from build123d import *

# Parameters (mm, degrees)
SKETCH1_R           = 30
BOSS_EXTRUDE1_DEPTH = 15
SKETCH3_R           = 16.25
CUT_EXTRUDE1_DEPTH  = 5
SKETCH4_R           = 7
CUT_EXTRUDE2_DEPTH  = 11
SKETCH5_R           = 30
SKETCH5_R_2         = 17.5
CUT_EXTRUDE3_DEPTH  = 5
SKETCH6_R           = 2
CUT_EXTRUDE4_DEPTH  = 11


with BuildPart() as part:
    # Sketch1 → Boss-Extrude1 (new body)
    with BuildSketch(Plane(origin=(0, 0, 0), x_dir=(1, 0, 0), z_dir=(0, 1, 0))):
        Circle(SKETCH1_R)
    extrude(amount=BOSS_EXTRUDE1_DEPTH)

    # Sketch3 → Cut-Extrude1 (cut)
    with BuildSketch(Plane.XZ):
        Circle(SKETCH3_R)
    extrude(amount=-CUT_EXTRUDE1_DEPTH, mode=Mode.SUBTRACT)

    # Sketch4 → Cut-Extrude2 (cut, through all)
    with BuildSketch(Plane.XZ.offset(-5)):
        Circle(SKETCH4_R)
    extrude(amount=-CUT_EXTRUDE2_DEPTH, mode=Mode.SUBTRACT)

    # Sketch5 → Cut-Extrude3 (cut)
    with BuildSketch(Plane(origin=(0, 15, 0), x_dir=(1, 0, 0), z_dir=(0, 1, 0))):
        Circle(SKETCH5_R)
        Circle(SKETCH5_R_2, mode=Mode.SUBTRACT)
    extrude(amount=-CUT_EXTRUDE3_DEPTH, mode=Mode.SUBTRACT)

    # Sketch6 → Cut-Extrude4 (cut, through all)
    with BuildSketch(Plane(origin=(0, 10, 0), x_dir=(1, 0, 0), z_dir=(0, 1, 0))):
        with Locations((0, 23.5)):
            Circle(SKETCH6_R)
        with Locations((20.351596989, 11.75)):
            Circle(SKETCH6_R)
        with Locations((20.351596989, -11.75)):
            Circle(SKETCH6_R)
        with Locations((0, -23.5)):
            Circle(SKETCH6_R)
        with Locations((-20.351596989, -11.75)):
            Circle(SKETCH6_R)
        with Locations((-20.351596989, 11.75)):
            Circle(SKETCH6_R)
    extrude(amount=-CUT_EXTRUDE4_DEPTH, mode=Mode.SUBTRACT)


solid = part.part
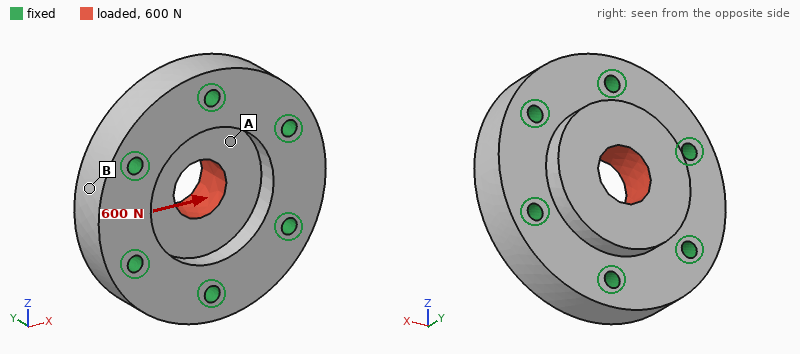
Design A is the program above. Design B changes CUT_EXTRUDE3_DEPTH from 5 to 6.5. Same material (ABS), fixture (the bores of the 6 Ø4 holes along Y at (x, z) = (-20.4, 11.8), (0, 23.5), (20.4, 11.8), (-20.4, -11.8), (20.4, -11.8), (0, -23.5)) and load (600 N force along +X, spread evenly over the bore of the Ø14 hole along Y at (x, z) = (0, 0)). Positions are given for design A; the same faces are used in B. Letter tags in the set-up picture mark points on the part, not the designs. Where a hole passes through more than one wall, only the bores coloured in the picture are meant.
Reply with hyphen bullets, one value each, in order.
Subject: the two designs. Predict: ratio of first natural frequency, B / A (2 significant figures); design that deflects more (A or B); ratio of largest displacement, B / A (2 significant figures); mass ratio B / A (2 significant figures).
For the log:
- 0.95
- B
- 1.2
- 0.90
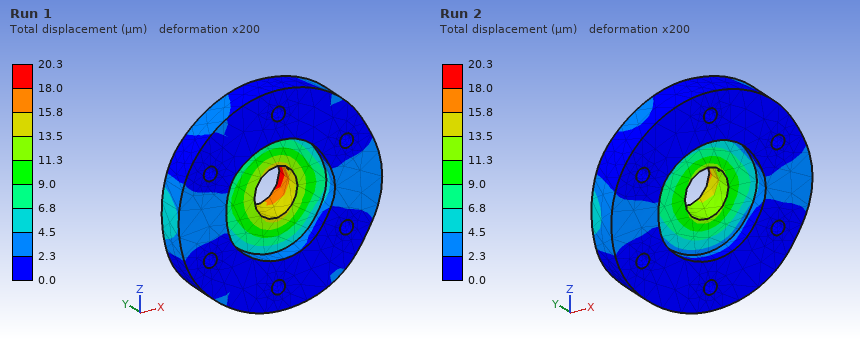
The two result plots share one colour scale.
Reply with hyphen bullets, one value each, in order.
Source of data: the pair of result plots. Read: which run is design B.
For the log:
- Run 1
